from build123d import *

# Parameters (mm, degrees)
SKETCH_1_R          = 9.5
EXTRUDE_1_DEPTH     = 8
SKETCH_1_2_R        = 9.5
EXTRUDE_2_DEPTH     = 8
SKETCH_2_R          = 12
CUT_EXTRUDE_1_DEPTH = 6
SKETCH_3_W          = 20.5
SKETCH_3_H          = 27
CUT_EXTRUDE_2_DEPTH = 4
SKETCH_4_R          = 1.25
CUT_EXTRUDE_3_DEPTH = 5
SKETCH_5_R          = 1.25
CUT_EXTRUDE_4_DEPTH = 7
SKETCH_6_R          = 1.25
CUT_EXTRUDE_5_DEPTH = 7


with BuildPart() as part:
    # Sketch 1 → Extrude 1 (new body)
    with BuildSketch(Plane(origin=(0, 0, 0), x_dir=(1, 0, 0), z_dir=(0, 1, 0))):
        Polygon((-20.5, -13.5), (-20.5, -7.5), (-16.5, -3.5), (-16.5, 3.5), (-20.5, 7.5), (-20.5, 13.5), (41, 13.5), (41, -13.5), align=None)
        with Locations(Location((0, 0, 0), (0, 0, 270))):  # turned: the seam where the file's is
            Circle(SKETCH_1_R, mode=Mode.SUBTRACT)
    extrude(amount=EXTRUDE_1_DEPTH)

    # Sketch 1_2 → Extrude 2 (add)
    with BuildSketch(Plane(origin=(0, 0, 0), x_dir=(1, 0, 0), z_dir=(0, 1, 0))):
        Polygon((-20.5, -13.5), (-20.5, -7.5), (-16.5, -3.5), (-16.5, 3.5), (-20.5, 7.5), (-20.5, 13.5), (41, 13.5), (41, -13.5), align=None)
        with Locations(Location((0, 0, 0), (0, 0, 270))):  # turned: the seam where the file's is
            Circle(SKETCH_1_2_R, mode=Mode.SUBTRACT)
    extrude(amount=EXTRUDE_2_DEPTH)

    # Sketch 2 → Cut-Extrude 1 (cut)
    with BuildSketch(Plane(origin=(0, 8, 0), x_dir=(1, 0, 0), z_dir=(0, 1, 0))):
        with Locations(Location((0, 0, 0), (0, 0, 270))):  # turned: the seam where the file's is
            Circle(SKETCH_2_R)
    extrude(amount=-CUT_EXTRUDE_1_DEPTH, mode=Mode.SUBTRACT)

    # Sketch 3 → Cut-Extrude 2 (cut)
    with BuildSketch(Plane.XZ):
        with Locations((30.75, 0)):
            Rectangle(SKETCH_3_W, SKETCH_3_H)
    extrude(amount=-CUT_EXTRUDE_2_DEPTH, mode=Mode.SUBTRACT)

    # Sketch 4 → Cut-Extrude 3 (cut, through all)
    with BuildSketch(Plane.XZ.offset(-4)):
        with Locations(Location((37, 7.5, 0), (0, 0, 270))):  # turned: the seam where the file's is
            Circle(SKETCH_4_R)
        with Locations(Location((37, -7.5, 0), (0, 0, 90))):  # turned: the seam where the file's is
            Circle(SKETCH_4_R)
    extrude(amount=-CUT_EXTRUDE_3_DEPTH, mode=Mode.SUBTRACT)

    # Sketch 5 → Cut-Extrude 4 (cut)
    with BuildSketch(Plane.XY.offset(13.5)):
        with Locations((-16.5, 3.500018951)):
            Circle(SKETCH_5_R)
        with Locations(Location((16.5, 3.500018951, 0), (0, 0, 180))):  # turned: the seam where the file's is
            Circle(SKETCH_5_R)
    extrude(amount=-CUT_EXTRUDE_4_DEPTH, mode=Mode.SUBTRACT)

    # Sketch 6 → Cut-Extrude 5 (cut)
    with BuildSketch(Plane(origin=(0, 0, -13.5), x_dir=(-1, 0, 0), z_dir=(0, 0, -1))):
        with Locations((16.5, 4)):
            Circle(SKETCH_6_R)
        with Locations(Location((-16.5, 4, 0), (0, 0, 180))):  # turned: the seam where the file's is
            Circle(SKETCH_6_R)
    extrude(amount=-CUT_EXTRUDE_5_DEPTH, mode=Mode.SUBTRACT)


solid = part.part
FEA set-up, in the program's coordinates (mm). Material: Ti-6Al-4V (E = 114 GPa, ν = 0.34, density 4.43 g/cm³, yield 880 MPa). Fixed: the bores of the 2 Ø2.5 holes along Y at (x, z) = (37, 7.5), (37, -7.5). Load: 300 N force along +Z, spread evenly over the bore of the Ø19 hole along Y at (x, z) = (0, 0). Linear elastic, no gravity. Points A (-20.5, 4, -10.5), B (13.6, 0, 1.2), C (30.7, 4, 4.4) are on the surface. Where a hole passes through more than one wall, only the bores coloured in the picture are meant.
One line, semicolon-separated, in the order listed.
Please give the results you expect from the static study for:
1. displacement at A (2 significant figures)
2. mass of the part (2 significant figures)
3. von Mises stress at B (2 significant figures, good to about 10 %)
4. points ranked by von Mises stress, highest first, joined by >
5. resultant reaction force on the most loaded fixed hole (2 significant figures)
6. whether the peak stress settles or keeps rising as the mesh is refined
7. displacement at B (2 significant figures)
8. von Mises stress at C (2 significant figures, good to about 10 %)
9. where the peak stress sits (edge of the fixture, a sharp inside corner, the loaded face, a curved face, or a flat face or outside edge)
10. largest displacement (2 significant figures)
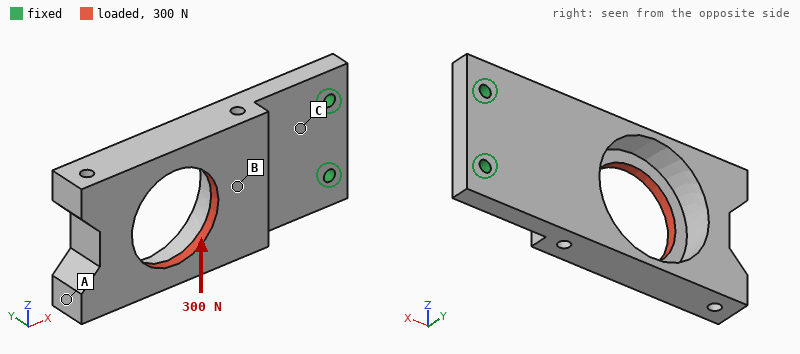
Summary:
31 µm; 32 g; 12 MPa; C > B > A; 690 N; keeps rising; 9.8 µm; 21 MPa; edge of the fixture; 33 µm
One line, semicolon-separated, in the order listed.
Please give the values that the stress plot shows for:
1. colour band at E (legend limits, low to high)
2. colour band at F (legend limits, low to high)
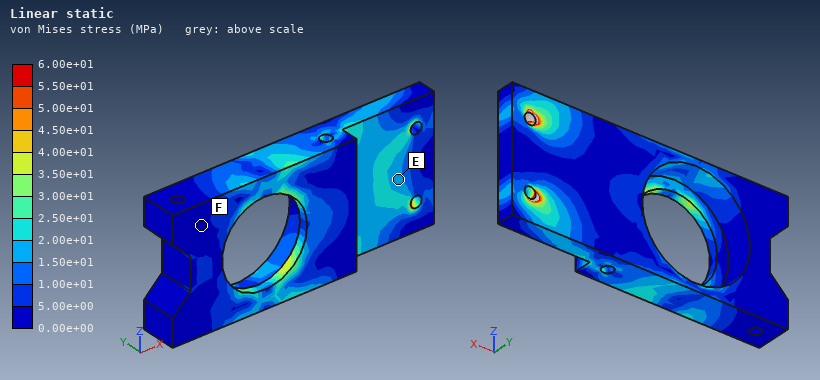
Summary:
1.50e+01 to 2.00e+01 MPa; 0.00e+00 to 5.00e+00 MPa
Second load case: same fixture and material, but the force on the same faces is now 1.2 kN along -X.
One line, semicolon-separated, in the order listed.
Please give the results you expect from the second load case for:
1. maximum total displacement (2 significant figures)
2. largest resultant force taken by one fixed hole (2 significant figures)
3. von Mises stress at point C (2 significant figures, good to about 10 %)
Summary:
0.36 mm; 600 N; 86 MPa
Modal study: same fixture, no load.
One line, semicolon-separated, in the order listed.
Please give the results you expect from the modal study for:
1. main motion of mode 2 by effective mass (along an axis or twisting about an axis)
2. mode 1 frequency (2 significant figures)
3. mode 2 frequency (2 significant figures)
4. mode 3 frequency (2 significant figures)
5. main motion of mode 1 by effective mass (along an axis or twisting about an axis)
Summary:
along Z; 990 Hz; 3600 Hz; 4200 Hz; along Y
